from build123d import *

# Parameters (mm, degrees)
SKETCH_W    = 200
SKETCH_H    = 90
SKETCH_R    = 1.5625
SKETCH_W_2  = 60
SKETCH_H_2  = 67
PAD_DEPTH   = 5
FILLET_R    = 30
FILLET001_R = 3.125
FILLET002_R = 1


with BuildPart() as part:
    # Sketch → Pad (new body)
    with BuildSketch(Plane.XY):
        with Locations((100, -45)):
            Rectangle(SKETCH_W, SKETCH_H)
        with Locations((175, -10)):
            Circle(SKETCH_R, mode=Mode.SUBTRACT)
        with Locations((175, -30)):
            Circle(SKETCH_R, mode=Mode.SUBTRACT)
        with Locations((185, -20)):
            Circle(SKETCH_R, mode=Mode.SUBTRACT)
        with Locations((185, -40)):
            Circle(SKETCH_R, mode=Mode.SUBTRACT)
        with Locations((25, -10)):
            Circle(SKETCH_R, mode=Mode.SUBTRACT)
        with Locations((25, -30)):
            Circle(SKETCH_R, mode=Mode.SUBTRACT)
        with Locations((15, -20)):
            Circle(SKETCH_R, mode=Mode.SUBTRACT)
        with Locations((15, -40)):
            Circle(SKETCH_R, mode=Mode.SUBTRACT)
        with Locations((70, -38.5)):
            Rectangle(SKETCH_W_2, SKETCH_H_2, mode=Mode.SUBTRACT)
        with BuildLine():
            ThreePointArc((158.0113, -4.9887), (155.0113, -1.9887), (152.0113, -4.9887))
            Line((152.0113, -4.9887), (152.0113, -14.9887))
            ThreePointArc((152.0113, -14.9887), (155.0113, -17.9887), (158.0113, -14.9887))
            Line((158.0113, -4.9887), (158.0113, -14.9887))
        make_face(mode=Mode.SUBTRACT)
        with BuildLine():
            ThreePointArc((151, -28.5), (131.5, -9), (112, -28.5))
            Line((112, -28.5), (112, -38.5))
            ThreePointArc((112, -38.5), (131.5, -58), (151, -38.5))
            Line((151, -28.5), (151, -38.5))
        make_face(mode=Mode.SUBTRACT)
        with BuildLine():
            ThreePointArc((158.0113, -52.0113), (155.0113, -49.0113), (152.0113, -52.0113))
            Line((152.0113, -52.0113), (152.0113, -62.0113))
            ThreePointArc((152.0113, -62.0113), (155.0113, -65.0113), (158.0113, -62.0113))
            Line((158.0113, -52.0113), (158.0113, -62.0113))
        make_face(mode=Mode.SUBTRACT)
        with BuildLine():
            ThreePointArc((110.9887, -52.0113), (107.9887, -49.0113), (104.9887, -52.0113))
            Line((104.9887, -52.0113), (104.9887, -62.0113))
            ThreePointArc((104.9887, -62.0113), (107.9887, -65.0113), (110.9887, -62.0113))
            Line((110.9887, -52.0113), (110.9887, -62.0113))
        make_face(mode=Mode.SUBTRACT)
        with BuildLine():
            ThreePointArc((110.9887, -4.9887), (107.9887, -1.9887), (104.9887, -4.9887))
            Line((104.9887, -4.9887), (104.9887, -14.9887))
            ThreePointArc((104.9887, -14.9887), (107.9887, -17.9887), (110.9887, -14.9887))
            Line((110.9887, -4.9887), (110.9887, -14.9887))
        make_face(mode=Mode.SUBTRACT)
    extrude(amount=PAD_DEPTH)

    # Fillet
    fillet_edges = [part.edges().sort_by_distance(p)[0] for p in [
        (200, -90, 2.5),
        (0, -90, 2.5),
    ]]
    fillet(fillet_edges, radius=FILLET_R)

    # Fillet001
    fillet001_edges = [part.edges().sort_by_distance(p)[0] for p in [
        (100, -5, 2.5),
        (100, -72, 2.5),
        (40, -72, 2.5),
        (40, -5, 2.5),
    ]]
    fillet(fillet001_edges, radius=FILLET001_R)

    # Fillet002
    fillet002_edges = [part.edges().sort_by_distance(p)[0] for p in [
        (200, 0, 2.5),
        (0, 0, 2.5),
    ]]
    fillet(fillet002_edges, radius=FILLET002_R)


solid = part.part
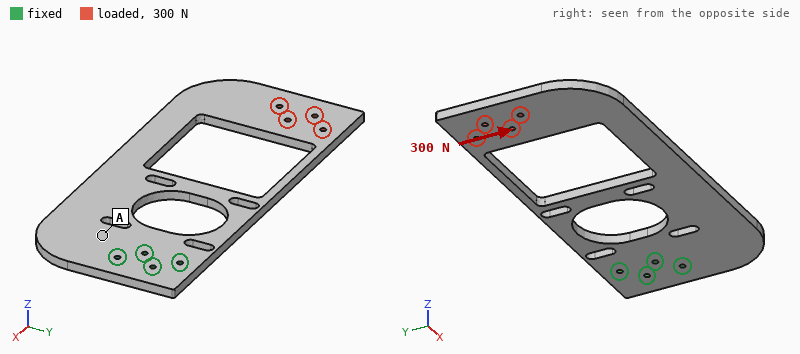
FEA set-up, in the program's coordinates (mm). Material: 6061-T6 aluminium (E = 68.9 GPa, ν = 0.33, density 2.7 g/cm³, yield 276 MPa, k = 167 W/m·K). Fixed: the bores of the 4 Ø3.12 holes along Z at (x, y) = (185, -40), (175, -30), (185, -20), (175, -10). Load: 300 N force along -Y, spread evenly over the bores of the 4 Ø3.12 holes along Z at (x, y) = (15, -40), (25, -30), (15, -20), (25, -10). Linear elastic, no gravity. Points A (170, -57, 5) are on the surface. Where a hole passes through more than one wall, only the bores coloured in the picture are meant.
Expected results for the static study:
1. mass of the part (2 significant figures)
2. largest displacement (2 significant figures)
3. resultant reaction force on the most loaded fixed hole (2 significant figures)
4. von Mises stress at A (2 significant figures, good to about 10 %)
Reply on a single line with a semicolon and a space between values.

160 g; 0.22 mm; 1.2 kN; 6.3 MPa
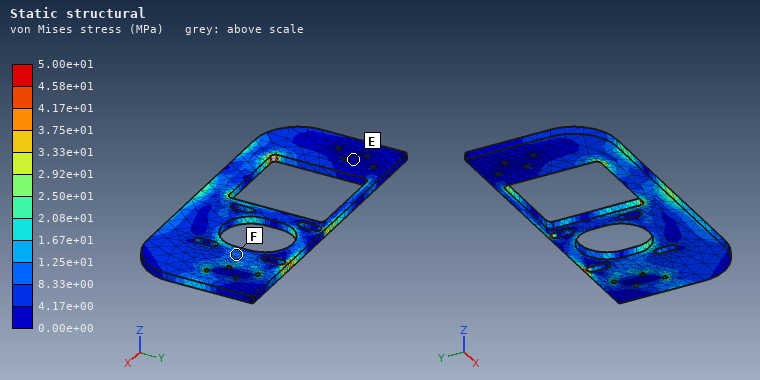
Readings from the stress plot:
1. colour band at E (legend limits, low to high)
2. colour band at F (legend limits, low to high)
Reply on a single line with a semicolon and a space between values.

0.00e+00 to 4.17e+00 MPa; 8.33e+00 to 1.25e+01 MPa
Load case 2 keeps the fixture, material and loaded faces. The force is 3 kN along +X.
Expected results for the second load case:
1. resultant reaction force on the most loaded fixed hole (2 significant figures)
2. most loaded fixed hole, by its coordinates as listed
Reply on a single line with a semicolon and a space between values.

1.3 kN; (175, -10)
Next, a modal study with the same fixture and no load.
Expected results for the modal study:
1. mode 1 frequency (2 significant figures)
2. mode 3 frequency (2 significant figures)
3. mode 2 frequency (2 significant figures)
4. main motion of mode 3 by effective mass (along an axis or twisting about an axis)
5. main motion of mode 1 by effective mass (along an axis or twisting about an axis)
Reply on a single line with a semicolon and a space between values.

99 Hz; 660 Hz; 360 Hz; along Z; along Z
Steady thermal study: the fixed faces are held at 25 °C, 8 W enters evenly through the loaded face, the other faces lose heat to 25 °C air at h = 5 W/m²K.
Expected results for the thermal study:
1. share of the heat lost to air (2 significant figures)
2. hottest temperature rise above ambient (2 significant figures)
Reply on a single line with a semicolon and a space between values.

31 %; 43 K
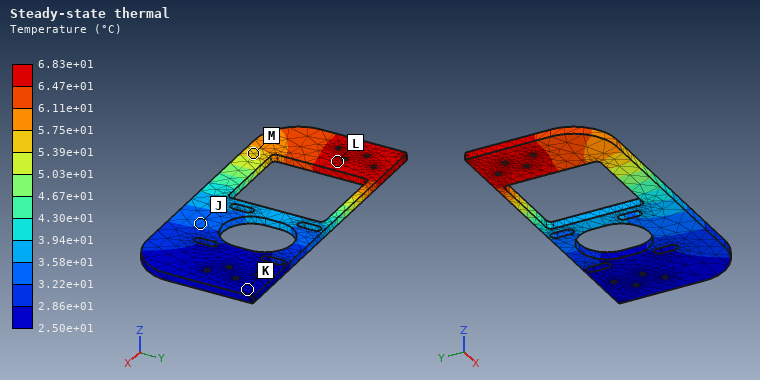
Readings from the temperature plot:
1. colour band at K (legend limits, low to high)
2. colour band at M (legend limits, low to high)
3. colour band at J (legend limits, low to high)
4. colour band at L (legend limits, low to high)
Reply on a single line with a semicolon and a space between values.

2.50e+01 to 2.86e+01 °C; 5.39e+01 to 5.75e+01 °C; 3.22e+01 to 3.58e+01 °C; 6.47e+01 to 6.83e+01 °C
